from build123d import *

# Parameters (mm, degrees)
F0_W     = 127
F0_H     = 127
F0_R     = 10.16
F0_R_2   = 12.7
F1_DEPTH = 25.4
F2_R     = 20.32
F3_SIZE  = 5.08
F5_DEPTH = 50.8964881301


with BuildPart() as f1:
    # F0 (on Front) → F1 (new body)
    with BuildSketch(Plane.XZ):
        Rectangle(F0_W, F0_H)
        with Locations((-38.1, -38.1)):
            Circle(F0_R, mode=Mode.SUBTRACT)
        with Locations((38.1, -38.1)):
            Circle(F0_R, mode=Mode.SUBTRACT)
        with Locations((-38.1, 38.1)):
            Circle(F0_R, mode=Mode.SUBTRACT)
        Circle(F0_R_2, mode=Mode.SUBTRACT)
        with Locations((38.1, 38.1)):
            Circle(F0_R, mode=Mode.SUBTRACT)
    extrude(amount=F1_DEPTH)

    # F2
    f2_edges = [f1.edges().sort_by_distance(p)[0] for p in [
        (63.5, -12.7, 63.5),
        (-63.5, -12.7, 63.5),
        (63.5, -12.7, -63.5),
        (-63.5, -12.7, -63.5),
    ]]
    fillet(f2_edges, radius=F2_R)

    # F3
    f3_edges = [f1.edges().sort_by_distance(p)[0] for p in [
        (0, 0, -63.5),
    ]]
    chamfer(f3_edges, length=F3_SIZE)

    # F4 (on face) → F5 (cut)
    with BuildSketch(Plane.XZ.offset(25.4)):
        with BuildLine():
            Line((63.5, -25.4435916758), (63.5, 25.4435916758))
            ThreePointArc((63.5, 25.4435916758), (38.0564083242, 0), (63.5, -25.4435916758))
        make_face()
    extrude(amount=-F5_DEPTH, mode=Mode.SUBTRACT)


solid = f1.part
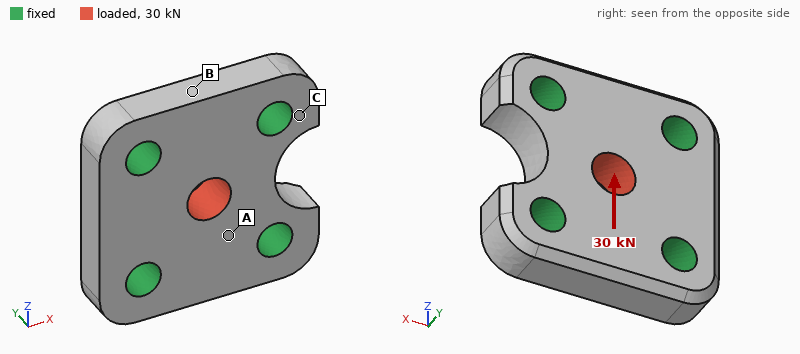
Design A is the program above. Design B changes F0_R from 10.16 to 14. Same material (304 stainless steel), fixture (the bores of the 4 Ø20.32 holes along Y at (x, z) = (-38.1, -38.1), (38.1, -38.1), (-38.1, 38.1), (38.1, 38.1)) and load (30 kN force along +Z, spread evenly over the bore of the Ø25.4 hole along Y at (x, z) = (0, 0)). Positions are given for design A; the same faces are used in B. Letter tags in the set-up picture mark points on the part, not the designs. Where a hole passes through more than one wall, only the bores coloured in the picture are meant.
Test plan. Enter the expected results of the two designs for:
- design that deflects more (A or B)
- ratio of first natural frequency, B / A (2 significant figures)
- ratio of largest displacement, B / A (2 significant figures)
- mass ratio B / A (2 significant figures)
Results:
A
1.2
0.87
0.91
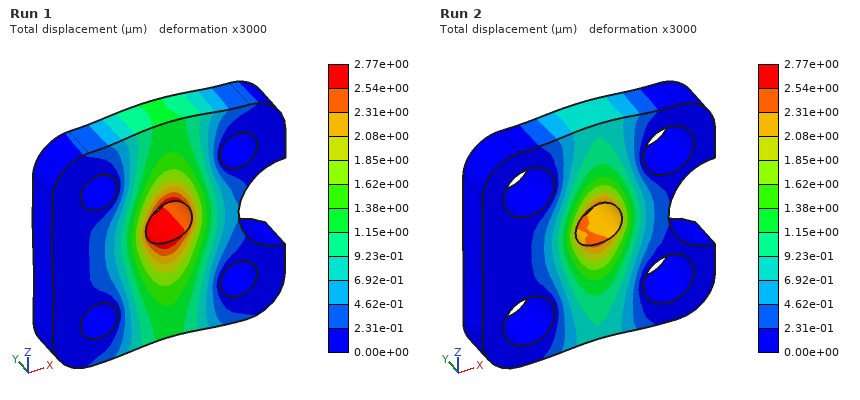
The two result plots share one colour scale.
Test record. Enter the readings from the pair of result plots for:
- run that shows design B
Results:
Run 2
